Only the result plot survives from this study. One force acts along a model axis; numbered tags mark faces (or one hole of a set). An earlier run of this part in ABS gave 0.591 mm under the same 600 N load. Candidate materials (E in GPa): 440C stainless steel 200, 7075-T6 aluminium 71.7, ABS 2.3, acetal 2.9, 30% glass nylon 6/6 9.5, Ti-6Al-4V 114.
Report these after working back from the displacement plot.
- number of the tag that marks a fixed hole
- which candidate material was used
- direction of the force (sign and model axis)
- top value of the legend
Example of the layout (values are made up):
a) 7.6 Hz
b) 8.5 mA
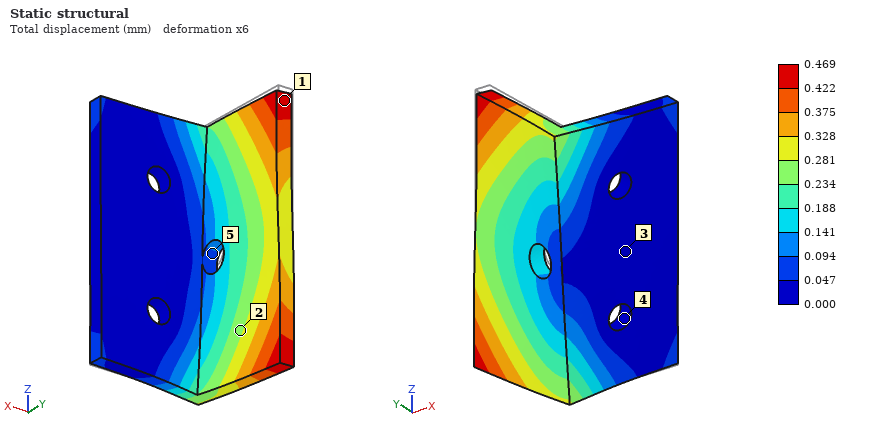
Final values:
a) 4
b) acetal
c) -Z
d) 0.469 mm
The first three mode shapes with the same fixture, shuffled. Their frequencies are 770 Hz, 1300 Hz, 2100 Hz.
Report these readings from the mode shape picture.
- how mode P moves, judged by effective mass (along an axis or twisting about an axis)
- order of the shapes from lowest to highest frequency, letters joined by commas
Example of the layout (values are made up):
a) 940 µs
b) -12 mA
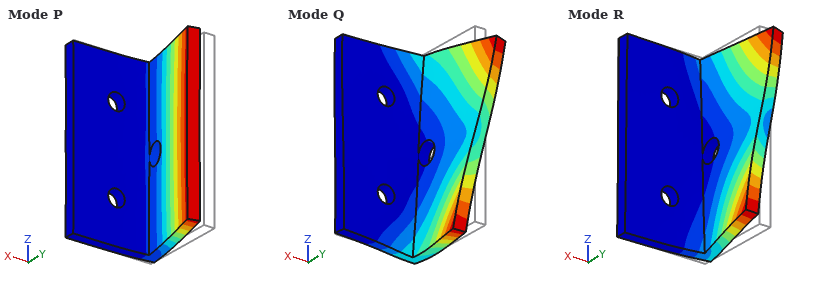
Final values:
a) along X
b) P, R, Q
